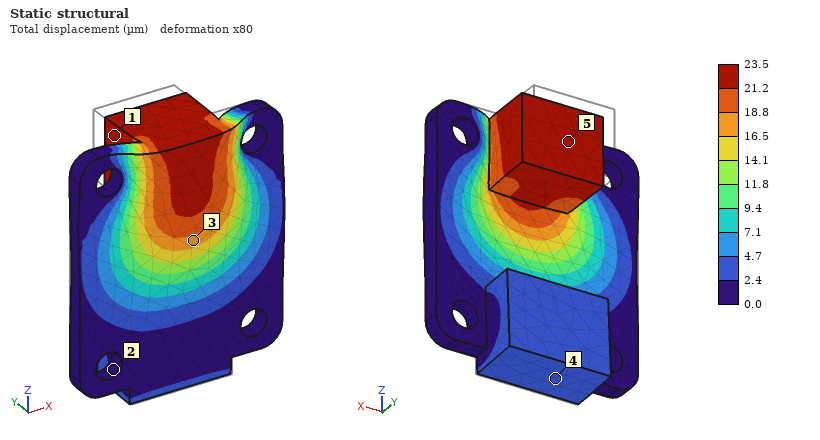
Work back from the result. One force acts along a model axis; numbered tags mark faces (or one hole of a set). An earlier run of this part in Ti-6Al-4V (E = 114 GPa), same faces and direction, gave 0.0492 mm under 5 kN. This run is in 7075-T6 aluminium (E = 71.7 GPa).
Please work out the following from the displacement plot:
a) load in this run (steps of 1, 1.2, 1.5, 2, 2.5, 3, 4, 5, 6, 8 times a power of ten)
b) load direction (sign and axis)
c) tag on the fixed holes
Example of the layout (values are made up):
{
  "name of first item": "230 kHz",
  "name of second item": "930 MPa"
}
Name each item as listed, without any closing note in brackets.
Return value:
{
  "load in this run": "1.5 kN",
  "load direction": "-Y",
  "tag on the fixed holes": "2"
}
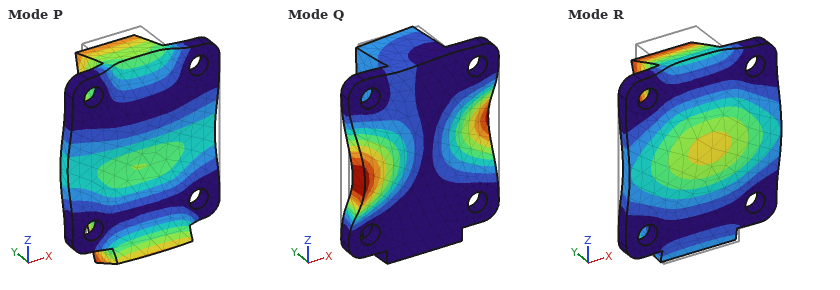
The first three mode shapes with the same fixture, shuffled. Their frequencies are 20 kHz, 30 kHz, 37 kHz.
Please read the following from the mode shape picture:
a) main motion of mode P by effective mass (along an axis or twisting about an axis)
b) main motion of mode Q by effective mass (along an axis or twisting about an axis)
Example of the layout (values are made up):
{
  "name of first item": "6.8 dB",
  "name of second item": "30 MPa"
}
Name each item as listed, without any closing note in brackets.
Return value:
{
  "main motion of mode P by effective mass": "along Z",
  "main motion of mode Q by effective mass": "twisting about Z"
}
